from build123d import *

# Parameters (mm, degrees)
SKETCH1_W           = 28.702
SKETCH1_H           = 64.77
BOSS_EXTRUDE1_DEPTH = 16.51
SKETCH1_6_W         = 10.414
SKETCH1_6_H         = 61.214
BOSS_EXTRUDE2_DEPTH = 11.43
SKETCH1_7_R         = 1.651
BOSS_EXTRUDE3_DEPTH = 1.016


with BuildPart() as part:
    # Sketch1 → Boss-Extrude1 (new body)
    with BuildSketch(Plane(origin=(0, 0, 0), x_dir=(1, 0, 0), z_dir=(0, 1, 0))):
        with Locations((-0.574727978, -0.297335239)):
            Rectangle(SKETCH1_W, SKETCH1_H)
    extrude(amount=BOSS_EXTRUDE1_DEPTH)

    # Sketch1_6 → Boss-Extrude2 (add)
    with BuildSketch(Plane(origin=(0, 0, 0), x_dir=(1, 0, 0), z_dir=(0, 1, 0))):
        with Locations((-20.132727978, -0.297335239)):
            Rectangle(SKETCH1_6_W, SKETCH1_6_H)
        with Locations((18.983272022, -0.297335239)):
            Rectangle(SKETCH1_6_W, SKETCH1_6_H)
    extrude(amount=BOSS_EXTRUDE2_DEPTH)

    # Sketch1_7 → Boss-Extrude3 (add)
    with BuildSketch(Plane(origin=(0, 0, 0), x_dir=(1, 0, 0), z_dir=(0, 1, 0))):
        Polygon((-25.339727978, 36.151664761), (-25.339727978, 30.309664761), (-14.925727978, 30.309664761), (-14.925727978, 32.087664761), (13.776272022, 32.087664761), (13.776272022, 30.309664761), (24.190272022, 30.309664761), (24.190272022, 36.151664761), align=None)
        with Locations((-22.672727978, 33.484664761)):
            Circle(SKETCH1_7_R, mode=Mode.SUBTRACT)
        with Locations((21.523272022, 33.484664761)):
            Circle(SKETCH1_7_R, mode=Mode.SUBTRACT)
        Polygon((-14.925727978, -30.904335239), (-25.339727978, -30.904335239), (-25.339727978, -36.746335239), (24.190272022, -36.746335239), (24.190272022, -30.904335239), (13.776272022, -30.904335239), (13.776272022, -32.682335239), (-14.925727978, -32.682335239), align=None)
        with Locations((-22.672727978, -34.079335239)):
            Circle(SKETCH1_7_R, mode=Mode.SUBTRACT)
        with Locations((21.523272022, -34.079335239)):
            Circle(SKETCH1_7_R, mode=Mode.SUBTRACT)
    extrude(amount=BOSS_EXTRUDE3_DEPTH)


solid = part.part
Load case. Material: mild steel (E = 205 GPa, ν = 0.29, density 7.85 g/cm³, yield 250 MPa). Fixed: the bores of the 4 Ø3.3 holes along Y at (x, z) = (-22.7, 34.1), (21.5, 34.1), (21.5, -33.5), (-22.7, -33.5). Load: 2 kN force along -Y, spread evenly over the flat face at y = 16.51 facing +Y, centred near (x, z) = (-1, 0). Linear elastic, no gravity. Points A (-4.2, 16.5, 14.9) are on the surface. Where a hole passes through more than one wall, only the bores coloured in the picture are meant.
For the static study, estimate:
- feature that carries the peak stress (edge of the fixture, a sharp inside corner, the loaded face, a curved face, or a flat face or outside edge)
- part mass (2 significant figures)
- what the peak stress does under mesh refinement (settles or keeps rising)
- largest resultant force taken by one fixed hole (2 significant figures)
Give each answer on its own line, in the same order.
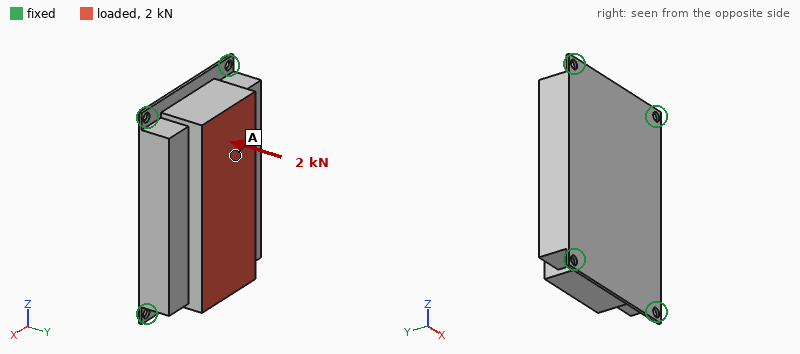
edge of the fixture
360 g
keeps rising
630 N
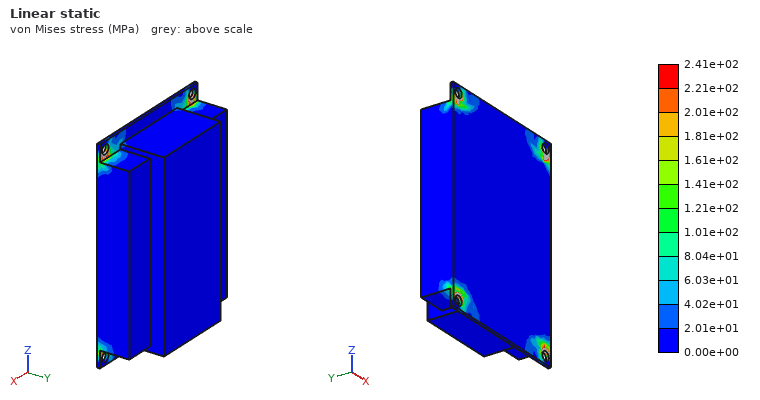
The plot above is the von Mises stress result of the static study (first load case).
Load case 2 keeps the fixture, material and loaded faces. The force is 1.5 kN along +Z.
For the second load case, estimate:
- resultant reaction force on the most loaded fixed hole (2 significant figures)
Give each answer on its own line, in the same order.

440 N
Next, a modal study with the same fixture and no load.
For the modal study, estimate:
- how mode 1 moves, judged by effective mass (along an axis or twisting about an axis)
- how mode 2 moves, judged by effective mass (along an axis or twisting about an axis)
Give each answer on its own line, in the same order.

along Y
along X
